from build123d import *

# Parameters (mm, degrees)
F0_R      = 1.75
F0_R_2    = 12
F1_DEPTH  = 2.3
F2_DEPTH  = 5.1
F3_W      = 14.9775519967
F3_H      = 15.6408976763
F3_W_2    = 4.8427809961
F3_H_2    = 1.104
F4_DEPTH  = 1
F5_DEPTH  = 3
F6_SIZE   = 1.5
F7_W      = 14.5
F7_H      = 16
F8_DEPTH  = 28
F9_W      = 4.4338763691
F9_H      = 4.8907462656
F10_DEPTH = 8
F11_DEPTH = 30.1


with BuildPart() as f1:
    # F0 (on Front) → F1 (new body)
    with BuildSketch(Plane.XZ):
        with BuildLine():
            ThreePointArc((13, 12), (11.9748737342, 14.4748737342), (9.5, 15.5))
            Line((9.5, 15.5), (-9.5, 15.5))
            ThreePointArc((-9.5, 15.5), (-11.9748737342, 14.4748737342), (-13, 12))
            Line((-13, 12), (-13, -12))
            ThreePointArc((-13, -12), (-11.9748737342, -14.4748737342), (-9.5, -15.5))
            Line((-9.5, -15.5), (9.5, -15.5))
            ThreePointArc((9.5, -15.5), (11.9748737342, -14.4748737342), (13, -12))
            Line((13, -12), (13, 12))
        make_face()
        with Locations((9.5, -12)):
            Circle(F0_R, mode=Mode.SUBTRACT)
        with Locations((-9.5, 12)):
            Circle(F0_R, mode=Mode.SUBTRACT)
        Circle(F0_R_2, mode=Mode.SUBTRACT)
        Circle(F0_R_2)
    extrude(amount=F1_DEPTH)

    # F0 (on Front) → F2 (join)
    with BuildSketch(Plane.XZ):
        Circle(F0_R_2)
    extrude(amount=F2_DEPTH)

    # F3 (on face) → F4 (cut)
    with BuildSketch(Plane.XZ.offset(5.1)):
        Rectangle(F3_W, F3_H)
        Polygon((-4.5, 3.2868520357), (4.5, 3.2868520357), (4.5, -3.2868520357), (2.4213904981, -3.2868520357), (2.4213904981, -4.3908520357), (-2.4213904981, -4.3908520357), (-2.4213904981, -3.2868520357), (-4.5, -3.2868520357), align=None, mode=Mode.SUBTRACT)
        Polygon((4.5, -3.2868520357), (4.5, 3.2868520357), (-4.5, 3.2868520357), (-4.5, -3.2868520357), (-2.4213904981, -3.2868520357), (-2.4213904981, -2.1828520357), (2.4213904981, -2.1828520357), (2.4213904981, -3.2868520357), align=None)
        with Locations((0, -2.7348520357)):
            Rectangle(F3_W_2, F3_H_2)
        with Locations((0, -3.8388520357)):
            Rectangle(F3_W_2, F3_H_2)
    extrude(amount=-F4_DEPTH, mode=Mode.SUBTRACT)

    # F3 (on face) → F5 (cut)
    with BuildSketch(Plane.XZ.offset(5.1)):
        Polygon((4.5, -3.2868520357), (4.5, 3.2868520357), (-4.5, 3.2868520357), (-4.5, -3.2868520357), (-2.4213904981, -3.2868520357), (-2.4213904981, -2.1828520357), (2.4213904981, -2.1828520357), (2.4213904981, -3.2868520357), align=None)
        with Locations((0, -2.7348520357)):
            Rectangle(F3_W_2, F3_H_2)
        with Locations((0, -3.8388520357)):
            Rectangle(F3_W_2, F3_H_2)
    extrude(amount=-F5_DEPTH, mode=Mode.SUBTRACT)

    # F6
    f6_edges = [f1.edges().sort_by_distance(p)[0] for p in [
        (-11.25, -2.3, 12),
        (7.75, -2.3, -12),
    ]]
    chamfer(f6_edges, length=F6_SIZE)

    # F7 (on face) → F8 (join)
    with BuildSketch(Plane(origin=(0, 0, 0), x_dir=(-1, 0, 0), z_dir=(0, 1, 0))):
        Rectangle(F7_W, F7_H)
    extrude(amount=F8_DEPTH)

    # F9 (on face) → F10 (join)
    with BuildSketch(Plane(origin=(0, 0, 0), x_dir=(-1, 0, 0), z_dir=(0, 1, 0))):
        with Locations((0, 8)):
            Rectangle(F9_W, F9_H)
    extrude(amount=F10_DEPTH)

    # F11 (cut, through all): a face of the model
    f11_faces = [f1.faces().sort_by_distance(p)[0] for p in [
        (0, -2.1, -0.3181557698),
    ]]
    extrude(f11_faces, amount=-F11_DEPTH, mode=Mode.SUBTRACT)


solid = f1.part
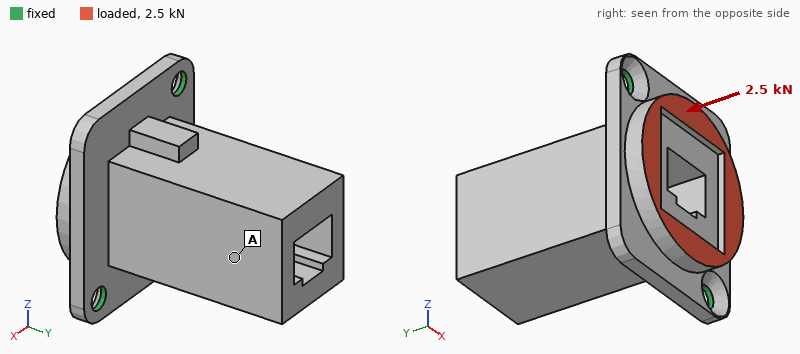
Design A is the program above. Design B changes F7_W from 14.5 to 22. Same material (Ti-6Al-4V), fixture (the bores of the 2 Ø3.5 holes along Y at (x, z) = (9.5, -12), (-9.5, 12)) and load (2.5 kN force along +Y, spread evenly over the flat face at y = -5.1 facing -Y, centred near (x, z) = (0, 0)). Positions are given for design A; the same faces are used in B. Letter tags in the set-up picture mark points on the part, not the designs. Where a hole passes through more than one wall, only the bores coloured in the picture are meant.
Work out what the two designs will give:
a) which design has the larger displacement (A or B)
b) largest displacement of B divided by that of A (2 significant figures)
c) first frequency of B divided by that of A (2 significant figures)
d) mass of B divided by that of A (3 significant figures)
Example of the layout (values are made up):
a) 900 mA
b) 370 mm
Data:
a) A
b) 0.66
c) 0.81
d) 1.46
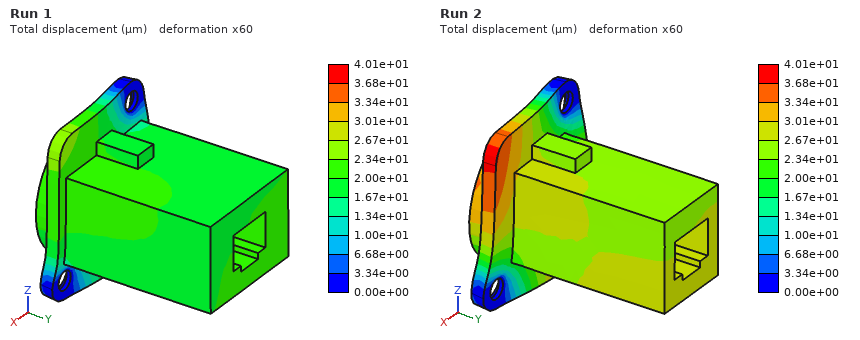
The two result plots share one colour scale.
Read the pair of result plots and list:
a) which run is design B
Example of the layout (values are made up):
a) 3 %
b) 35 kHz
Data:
a) Run 1
